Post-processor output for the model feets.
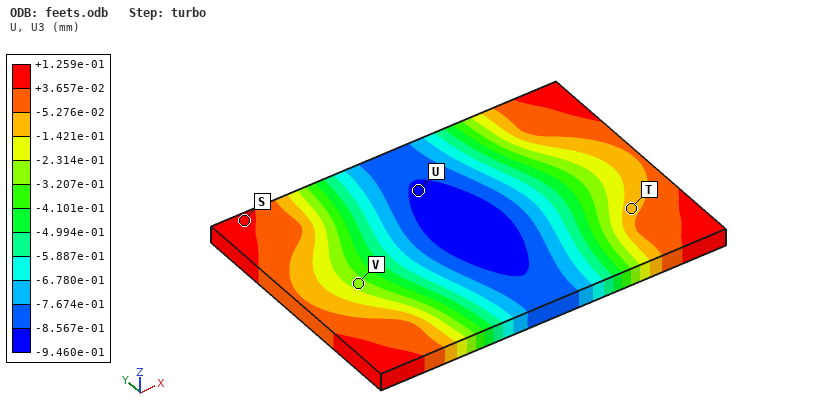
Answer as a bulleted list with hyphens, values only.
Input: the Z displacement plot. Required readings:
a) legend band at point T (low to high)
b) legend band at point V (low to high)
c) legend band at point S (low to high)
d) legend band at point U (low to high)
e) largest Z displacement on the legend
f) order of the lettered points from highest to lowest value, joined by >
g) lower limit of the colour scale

- -1.421e-01 to -5.276e-02 mm
- -3.207e-01 to -2.314e-01 mm
- +3.657e-02 to +1.259e-01 mm
- -9.460e-01 to -8.567e-01 mm
- +1.259e-01 mm
- S > T > V > U
- -9.460e-01 mm
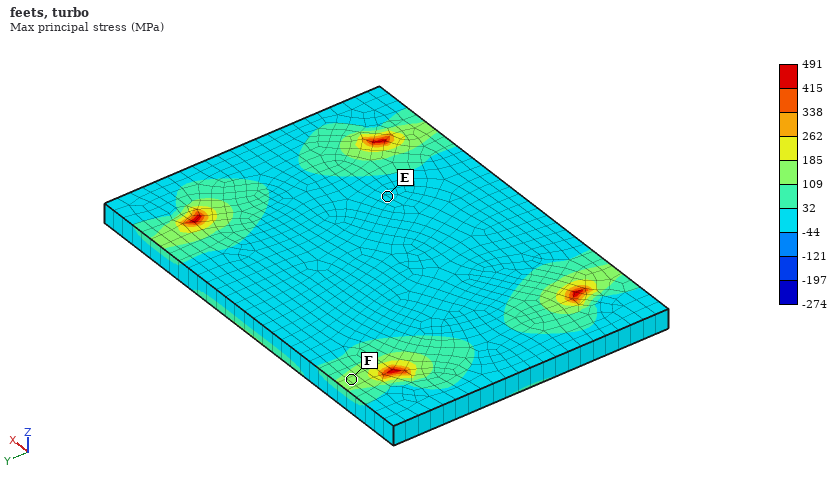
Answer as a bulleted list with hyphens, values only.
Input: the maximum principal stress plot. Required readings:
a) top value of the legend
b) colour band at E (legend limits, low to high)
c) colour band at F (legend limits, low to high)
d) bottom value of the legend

- 491 MPa
- -44 to 32 MPa
- 109 to 185 MPa
- -274 MPa
